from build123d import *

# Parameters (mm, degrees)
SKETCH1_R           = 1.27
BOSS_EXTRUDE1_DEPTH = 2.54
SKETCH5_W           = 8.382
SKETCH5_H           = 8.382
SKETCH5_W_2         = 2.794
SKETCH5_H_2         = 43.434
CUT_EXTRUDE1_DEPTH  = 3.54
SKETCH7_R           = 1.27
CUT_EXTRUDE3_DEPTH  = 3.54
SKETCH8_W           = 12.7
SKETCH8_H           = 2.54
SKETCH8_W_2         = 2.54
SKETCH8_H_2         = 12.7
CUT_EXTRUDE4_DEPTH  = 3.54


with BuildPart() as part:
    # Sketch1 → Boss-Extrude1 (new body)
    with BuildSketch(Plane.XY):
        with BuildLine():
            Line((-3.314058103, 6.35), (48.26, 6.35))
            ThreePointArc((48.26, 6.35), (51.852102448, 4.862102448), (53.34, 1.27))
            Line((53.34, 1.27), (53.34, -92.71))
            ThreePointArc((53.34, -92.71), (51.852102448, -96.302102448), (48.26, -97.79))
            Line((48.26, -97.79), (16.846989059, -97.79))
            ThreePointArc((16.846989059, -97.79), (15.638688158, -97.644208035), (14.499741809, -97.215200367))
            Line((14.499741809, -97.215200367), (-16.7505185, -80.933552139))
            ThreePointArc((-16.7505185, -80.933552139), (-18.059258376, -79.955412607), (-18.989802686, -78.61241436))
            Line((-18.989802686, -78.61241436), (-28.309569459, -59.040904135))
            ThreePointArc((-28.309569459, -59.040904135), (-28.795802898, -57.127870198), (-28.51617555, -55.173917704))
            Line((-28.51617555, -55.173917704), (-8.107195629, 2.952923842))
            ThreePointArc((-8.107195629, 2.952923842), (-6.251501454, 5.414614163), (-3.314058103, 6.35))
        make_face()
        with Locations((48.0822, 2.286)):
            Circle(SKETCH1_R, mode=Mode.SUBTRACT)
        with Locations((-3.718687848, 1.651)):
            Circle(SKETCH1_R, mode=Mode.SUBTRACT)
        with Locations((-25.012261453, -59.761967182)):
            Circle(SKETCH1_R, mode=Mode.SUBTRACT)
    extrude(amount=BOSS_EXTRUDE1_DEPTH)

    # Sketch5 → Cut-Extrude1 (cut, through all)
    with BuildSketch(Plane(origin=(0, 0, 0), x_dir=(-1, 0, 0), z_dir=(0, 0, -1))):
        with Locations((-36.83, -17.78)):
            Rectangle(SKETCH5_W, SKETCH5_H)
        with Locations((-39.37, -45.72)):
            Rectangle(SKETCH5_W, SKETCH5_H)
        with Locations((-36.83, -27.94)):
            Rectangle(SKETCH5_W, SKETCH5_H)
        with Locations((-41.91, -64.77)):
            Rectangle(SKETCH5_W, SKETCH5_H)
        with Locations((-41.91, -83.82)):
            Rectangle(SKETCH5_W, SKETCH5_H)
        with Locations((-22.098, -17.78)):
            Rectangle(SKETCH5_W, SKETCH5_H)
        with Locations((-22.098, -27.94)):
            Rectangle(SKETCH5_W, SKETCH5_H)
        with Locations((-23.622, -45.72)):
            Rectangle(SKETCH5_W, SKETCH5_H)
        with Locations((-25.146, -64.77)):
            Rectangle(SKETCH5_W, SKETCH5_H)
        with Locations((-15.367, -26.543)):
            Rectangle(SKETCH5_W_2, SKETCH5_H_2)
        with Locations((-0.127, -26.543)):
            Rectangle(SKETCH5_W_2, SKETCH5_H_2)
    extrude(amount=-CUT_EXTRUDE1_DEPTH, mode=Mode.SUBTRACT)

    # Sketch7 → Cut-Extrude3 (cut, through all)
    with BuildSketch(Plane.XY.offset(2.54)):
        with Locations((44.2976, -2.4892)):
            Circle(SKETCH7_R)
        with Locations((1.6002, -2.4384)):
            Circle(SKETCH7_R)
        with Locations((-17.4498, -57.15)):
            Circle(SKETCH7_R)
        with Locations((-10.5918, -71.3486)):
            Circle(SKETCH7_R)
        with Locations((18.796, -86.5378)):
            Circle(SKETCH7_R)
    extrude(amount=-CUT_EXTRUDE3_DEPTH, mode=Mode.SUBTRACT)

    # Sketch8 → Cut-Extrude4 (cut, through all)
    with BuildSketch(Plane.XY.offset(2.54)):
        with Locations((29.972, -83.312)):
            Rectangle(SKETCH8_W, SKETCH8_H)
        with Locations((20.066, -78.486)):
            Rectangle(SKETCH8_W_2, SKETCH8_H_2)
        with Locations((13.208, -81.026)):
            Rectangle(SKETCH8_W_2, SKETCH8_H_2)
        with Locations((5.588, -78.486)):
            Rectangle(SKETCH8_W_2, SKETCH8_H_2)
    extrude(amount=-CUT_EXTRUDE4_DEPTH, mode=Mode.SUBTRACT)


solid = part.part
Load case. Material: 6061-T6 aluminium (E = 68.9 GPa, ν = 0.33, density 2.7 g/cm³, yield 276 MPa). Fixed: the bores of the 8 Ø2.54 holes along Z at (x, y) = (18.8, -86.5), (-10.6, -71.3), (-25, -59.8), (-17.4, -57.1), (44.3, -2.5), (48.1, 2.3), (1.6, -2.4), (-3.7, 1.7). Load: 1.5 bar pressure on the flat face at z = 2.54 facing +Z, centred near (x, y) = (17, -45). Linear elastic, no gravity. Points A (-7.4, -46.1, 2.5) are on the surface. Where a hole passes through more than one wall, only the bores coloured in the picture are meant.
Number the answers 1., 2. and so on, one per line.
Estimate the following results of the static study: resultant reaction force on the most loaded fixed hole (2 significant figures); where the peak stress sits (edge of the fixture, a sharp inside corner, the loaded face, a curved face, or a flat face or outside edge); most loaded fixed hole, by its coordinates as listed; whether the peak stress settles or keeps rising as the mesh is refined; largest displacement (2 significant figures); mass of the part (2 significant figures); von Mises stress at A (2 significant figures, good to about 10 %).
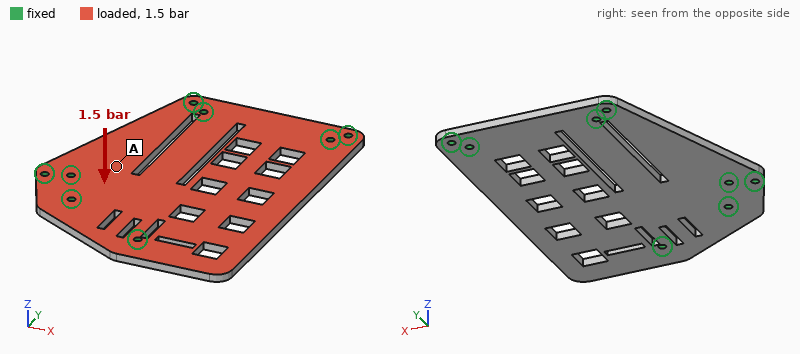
1. 370 N
2. edge of the fixture
3. (44.3, -2.5)
4. keeps rising
5. 0.61 mm
6. 43 g
7. 23 MPa
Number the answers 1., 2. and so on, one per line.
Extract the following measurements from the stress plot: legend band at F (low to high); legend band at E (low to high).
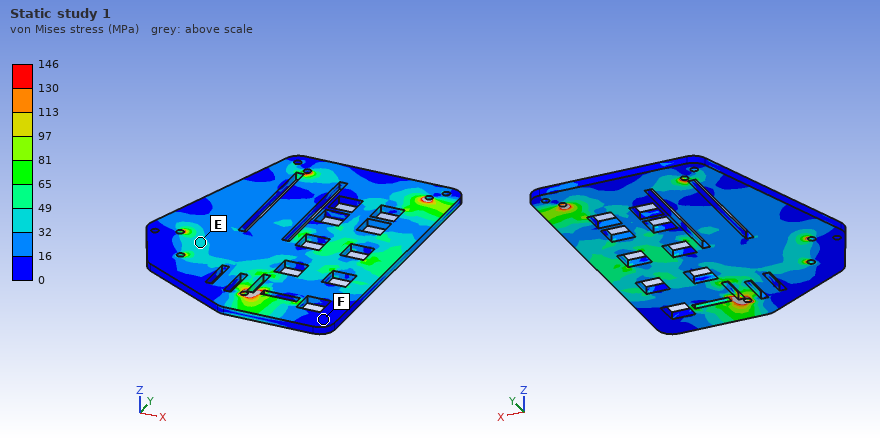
1. 0 to 16 MPa
2. 32 to 49 MPa
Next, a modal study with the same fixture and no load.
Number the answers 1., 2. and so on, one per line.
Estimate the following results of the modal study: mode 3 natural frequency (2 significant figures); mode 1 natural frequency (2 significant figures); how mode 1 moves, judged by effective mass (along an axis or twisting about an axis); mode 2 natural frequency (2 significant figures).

1. 3100 Hz
2. 1200 Hz
3. along Z
4. 2200 Hz
